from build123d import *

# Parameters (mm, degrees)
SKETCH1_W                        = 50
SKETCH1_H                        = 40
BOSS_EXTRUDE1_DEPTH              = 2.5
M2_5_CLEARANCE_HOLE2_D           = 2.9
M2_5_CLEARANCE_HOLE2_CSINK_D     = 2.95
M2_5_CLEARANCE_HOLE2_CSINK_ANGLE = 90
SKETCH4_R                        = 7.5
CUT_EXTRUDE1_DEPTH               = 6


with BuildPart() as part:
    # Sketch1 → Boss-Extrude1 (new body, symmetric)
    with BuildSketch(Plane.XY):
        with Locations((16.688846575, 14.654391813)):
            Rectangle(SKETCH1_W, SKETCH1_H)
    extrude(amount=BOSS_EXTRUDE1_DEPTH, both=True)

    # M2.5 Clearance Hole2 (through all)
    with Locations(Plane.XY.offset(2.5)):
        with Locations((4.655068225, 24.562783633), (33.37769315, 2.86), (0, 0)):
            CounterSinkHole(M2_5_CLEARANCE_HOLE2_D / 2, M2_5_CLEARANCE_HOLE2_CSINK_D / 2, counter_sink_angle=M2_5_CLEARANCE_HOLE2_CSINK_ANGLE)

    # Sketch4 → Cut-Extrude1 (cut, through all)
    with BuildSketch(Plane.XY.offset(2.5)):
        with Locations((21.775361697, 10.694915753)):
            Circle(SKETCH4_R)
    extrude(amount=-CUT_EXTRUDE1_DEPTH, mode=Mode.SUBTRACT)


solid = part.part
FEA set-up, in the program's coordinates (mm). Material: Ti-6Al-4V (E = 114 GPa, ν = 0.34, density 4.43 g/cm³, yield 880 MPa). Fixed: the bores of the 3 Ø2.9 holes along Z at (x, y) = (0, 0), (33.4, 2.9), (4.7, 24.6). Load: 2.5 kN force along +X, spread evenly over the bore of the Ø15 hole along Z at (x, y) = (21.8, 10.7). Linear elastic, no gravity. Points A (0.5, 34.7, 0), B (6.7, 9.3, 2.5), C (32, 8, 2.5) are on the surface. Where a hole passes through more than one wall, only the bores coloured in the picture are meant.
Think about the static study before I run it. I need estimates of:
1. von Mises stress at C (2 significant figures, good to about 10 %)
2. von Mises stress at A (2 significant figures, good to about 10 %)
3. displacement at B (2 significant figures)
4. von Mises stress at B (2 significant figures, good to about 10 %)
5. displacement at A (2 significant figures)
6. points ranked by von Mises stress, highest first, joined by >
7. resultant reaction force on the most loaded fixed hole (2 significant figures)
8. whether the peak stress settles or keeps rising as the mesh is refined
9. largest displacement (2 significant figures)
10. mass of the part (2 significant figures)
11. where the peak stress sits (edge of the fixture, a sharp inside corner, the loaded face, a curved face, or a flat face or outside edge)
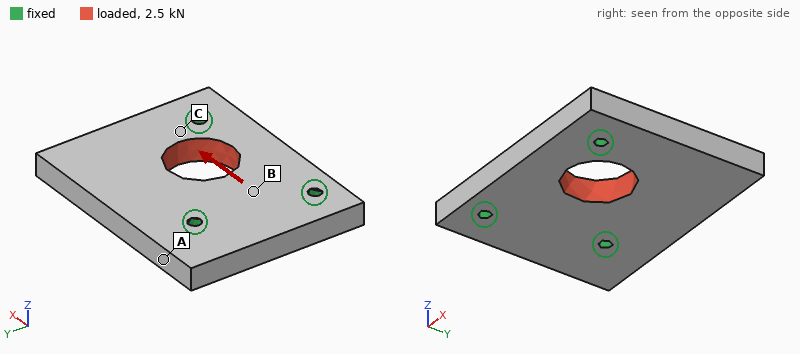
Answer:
13 MPa
3.5 MPa
1.2 µm
7.6 MPa
0.61 µm
C > B > A
970 N
keeps rising
2.9 µm
40 g
edge of the fixture
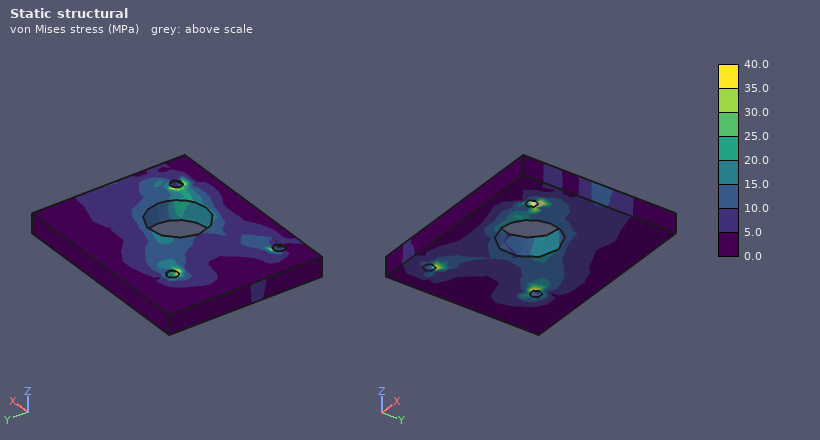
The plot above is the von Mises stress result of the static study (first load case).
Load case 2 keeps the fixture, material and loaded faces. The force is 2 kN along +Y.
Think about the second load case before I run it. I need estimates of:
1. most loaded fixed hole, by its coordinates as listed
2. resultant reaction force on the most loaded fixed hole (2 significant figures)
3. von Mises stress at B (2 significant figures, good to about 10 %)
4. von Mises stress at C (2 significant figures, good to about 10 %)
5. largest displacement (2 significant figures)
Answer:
(33.4, 2.9)
1.0 kN
9.3 MPa
22 MPa
2.9 µm
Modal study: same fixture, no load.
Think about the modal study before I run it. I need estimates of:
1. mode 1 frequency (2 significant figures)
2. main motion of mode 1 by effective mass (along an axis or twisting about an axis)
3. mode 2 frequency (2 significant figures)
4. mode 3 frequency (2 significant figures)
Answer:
5800 Hz
along Z
17 kHz
20 kHz
